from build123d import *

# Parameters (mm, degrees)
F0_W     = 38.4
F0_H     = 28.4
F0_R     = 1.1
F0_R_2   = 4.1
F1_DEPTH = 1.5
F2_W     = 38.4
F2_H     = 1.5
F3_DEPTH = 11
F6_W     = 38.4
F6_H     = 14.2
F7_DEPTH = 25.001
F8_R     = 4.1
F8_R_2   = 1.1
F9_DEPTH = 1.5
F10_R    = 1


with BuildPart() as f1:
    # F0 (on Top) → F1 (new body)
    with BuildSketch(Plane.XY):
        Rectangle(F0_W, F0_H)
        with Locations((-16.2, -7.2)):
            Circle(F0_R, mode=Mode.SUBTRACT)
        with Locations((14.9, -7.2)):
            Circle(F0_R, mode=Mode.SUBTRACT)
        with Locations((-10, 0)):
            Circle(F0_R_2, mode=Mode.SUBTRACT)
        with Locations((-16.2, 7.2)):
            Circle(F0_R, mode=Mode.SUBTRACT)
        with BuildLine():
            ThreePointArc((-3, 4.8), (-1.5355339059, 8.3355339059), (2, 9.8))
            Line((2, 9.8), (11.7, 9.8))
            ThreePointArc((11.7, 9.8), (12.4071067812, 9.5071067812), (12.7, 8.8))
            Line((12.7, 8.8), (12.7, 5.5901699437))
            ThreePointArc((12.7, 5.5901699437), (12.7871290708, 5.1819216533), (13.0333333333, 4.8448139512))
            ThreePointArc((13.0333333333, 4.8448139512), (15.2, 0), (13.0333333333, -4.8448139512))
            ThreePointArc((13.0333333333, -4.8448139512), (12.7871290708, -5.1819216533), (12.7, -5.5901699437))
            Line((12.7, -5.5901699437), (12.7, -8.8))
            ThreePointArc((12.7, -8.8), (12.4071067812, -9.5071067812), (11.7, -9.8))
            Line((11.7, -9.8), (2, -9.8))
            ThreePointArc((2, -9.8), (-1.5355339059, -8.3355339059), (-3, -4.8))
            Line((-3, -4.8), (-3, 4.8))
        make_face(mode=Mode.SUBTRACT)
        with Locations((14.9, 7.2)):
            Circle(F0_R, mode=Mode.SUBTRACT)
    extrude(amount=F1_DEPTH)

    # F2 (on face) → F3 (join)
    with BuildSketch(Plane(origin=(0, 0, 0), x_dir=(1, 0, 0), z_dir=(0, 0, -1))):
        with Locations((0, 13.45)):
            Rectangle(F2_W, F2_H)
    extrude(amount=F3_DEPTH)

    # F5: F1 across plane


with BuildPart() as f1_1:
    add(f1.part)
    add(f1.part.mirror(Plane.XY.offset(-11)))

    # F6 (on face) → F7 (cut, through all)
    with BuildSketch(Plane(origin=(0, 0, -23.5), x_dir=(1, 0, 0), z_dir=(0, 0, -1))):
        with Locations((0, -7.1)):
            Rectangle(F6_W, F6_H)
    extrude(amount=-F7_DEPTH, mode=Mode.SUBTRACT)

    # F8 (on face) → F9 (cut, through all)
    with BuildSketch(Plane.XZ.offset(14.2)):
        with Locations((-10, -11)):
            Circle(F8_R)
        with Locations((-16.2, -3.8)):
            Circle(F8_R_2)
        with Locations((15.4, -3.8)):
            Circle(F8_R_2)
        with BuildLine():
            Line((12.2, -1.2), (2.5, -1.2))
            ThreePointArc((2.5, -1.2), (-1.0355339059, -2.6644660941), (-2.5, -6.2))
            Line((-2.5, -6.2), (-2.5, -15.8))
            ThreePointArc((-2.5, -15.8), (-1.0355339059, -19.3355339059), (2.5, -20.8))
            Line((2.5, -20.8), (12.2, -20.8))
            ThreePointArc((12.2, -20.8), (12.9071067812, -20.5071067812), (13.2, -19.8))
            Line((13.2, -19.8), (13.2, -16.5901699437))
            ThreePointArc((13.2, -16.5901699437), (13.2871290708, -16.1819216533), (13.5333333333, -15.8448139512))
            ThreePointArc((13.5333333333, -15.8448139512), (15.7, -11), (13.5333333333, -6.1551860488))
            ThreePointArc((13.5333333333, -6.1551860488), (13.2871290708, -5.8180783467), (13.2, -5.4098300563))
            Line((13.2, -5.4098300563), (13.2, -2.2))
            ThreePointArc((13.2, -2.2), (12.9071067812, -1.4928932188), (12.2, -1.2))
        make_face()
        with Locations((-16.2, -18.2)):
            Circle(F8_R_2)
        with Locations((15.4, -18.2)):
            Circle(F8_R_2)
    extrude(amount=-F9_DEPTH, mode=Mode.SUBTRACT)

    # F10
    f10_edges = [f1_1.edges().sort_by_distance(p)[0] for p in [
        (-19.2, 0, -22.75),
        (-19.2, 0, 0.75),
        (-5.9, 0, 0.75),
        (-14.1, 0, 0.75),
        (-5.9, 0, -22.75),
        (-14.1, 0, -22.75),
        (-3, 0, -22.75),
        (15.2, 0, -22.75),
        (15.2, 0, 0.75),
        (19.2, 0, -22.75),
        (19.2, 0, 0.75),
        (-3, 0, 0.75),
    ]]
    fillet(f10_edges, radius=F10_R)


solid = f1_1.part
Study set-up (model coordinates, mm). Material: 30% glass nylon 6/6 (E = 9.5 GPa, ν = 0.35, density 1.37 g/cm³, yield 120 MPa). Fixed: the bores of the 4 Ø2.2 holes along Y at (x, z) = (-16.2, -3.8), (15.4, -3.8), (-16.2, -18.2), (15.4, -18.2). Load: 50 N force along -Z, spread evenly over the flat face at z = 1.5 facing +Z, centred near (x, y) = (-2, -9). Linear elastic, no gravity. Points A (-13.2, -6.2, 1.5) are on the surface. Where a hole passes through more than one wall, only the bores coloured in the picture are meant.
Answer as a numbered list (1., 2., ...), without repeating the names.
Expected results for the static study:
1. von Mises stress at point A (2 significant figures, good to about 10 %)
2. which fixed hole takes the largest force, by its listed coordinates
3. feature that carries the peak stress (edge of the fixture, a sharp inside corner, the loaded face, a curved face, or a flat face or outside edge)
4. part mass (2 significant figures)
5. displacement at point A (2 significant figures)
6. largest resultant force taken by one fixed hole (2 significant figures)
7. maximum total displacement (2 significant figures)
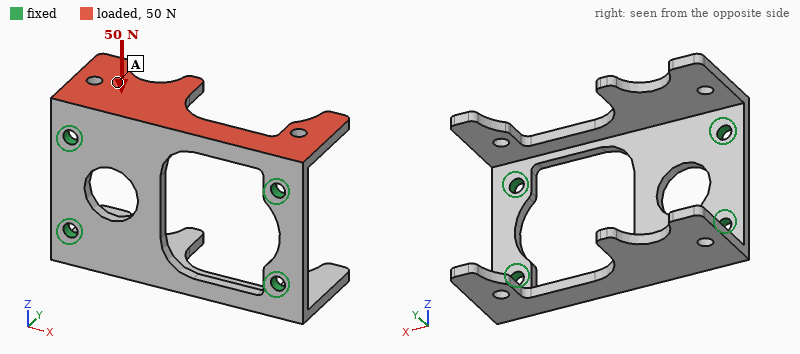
1. 5.2 MPa
2. (-16.2, -3.8)
3. a flat face or outside edge
4. 2.4 g
5. 0.19 mm
6. 25 N
7. 0.37 mm
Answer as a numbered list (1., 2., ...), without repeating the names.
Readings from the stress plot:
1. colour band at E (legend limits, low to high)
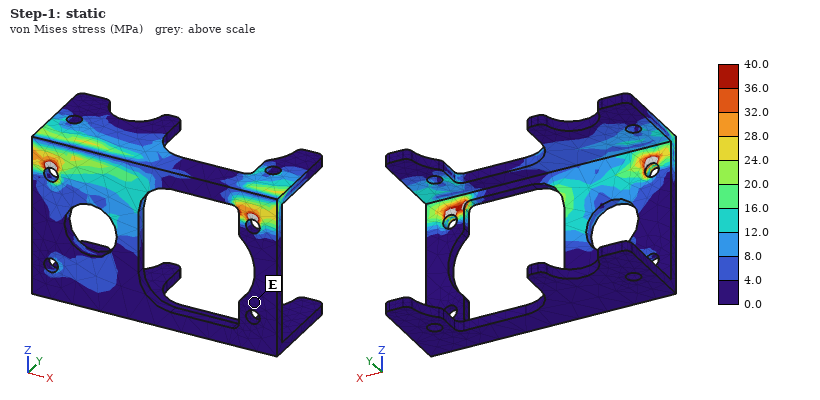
1. 0.0 to 4.0 MPa
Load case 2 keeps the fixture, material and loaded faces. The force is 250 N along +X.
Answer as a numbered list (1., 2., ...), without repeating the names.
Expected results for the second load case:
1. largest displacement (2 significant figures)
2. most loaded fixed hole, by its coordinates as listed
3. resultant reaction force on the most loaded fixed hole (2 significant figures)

1. 0.19 mm
2. (-16.2, -3.8)
3. 180 N
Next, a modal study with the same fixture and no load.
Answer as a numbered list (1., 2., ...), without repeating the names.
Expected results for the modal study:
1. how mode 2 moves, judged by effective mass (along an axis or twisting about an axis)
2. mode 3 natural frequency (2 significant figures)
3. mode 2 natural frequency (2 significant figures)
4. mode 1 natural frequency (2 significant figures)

1. along Z
2. 3200 Hz
3. 2800 Hz
4. 2700 Hz
